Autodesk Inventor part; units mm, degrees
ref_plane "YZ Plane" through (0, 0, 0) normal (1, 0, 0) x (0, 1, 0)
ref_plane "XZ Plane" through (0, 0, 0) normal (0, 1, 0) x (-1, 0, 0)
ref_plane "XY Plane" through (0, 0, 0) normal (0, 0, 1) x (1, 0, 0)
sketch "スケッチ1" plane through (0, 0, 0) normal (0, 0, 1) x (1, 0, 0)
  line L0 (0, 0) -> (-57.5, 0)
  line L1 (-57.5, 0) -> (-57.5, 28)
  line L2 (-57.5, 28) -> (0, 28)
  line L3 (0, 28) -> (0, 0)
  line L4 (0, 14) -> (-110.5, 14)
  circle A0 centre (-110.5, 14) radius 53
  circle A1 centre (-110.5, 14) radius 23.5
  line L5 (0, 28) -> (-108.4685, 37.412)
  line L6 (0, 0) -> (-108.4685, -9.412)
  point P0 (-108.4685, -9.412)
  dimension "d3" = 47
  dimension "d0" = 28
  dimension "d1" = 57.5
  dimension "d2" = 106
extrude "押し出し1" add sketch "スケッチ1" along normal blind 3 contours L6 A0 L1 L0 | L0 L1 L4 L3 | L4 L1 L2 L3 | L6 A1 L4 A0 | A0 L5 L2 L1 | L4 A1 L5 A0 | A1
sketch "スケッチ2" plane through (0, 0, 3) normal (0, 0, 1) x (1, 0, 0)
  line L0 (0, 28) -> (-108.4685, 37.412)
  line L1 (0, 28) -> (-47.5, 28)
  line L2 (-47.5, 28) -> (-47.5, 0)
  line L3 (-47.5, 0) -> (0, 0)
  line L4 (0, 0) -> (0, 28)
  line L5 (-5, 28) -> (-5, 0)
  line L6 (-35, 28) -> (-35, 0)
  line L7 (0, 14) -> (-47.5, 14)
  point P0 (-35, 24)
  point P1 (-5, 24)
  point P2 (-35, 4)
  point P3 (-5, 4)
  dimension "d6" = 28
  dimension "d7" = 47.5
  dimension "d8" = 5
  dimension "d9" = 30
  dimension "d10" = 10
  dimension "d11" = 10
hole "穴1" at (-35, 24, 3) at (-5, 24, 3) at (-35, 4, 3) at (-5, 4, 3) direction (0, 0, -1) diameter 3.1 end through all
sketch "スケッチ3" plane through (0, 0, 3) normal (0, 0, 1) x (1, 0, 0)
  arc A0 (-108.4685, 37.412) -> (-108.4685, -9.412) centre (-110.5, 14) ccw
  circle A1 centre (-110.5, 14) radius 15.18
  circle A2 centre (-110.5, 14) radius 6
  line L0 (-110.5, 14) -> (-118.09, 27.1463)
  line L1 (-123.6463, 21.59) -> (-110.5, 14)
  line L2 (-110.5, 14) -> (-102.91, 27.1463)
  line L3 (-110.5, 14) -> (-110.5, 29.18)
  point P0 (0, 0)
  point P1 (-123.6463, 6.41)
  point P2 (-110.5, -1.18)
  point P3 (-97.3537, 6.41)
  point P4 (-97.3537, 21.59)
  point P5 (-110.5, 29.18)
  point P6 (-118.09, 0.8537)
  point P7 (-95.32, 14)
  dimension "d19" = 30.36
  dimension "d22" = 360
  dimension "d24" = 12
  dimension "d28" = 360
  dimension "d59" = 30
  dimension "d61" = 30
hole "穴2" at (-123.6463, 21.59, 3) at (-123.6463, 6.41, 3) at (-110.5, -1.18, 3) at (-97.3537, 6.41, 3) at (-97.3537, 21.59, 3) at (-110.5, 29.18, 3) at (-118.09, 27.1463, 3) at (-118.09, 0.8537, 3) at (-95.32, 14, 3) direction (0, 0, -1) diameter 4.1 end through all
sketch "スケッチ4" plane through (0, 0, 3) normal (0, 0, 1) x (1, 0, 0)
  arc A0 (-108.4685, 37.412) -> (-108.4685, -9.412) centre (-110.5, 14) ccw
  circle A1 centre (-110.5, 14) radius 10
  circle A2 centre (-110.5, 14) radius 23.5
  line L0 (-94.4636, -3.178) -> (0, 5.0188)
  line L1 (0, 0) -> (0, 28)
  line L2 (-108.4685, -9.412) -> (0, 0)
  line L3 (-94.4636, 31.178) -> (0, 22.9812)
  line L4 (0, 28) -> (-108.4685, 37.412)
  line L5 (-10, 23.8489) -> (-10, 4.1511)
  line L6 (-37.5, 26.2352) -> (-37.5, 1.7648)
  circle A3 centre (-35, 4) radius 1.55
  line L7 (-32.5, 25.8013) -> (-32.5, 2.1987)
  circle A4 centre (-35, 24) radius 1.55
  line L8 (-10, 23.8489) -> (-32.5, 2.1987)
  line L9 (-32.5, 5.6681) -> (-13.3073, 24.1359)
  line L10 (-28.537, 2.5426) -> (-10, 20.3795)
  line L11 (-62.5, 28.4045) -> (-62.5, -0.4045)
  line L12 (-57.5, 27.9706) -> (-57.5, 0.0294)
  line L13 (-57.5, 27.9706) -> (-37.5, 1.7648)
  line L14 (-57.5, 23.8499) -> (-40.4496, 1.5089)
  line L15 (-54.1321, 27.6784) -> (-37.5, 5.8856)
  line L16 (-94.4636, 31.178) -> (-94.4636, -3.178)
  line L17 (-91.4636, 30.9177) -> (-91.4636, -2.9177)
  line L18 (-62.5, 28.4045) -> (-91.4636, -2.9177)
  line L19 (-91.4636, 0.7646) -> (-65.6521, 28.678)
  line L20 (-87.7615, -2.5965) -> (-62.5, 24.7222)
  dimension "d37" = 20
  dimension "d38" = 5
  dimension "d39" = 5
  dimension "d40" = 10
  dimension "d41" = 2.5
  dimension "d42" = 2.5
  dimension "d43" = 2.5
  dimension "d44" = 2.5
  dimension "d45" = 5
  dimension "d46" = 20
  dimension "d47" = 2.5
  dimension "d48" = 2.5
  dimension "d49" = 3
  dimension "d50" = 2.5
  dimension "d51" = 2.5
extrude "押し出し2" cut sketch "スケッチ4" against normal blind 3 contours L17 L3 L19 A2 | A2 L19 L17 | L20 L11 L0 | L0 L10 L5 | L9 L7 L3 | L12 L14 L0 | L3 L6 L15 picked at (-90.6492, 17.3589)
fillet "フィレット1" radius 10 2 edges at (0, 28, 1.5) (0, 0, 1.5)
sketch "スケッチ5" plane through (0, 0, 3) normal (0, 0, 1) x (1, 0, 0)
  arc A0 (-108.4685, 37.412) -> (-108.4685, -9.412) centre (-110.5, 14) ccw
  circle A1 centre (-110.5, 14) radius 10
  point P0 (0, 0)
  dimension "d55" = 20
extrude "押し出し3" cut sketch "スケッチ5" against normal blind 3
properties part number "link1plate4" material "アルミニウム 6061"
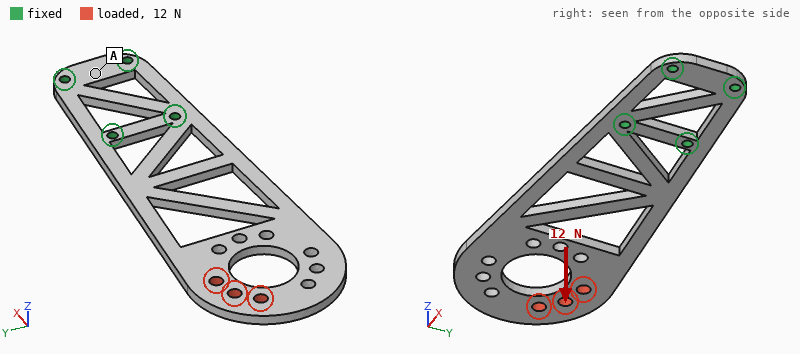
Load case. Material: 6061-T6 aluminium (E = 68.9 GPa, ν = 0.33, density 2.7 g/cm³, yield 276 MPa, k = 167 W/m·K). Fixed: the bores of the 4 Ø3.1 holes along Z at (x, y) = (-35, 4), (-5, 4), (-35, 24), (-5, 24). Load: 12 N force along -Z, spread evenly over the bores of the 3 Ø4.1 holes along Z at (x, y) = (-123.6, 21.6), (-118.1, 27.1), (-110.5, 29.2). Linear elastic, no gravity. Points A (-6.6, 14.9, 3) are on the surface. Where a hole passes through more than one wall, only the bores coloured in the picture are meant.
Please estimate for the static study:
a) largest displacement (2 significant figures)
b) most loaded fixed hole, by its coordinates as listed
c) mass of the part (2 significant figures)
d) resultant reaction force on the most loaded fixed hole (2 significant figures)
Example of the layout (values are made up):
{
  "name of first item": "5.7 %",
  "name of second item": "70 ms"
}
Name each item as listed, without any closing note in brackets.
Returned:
{
  "largest displacement": "1.4 mm",
  "most loaded fixed hole, by its coordinates as listed": "(-35, 24)",
  "mass of the part": "25 g",
  "resultant reaction force on the most loaded fixed hole": "9.2 N"
}
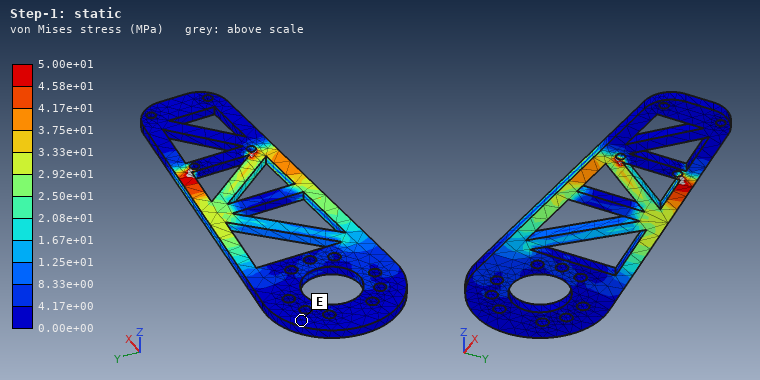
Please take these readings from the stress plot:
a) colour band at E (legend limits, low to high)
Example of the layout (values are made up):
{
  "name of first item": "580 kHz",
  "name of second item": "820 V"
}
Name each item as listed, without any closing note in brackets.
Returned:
{
  "colour band at E": "0.00e+00 to 4.17e+00 MPa"
}
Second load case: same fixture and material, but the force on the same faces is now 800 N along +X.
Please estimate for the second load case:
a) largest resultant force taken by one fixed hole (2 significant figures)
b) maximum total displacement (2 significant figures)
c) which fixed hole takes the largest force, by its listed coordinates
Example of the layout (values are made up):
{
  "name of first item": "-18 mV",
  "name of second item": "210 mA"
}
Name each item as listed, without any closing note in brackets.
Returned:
{
  "largest resultant force taken by one fixed hole": "510 N",
  "maximum total displacement": "0.10 mm",
  "which fixed hole takes the largest force, by its listed coordinates": "(-35, 24)"
}
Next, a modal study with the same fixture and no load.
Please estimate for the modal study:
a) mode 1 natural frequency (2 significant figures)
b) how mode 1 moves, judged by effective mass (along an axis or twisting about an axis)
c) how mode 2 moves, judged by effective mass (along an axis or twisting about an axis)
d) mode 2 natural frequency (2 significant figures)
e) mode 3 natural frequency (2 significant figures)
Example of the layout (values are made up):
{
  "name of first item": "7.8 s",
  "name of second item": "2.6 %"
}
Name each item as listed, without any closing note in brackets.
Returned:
{
  "mode 1 natural frequency": "180 Hz",
  "how mode 1 moves, judged by effective mass": "along Z",
  "how mode 2 moves, judged by effective mass": "twisting about X",
  "mode 2 natural frequency": "800 Hz",
  "mode 3 natural frequency": "1300 Hz"
}
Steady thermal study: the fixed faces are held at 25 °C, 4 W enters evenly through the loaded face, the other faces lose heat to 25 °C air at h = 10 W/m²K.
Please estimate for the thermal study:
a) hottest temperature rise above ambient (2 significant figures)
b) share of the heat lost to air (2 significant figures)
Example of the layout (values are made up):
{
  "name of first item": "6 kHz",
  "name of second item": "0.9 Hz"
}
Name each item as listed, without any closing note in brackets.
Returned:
{
  "hottest temperature rise above ambient": "34 K",
  "share of the heat lost to air": "34 %"
}
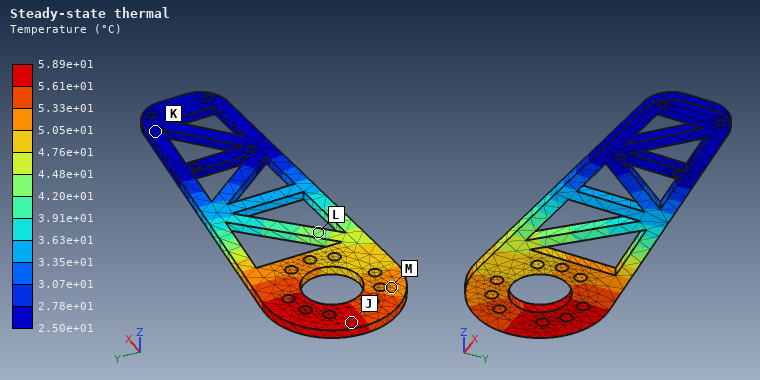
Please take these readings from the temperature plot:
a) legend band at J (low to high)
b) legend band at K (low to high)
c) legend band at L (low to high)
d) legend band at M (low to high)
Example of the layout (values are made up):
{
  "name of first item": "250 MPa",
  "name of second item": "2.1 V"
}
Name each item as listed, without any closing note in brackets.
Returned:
{
  "legend band at J": "5.61e+01 to 5.89e+01 °C",
  "legend band at K": "2.50e+01 to 2.78e+01 °C",
  "legend band at L": "4.20e+01 to 4.48e+01 °C",
  "legend band at M": "5.05e+01 to 5.33e+01 °C"
}
